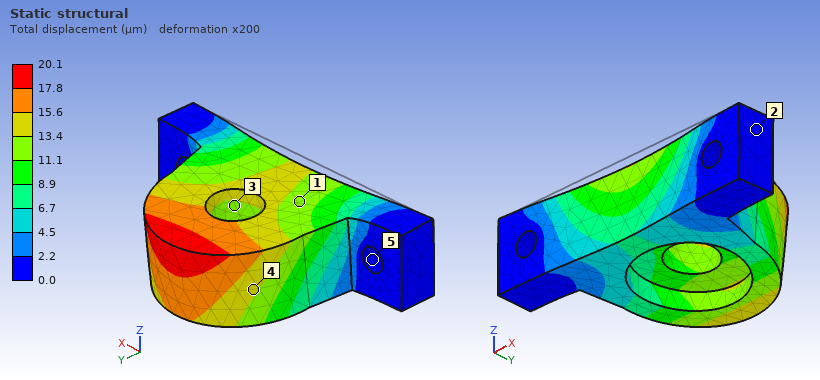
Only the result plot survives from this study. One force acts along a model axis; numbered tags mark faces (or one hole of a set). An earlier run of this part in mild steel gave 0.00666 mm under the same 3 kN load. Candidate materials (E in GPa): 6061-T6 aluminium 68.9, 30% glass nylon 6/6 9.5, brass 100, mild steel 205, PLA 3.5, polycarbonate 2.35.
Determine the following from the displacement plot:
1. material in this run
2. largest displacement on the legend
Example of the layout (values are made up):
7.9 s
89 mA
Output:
6061-T6 aluminium
20.1 µm
